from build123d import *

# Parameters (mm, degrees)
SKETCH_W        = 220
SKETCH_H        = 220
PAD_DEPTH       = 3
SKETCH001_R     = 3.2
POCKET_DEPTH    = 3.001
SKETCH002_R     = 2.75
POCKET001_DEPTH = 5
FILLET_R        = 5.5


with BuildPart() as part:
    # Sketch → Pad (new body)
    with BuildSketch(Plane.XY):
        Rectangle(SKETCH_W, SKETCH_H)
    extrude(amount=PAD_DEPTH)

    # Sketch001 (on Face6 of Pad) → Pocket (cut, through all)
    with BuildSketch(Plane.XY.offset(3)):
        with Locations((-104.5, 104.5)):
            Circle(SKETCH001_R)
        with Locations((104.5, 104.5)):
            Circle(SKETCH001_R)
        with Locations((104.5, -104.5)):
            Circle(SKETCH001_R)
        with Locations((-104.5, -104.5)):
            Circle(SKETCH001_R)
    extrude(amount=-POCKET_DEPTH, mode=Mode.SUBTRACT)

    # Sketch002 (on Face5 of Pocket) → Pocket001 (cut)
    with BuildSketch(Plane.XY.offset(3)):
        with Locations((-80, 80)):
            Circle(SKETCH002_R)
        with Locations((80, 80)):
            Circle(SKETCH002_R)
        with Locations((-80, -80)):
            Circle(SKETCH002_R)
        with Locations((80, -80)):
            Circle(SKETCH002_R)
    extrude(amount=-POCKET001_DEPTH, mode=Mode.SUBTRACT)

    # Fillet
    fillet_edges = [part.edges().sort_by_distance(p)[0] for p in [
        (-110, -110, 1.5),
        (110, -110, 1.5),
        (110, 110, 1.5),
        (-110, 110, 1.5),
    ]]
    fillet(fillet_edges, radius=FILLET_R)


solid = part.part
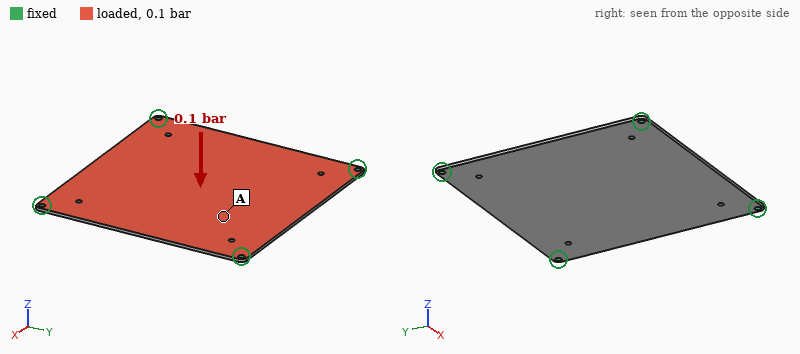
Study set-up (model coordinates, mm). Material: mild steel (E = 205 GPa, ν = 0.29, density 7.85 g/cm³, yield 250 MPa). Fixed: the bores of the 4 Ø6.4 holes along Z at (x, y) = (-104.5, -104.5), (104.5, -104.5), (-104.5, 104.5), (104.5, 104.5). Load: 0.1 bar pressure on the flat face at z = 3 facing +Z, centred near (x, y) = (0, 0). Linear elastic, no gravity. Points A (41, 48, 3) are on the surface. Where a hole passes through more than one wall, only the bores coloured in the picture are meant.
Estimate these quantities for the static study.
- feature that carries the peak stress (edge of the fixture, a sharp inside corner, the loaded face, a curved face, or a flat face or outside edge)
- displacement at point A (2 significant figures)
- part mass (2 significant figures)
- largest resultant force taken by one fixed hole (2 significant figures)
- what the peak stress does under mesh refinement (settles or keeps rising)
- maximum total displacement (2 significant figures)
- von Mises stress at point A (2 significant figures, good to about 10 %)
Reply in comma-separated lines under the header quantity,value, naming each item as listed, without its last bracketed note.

quantity,value
feature that carries the peak stress,edge of the fixture
displacement at point A,0.28 mm
part mass,1.1 kg
largest resultant force taken by one fixed hole,120 N
what the peak stress does under mesh refinement,keeps rising
maximum total displacement,0.37 mm
von Mises stress at point A,14 MPa
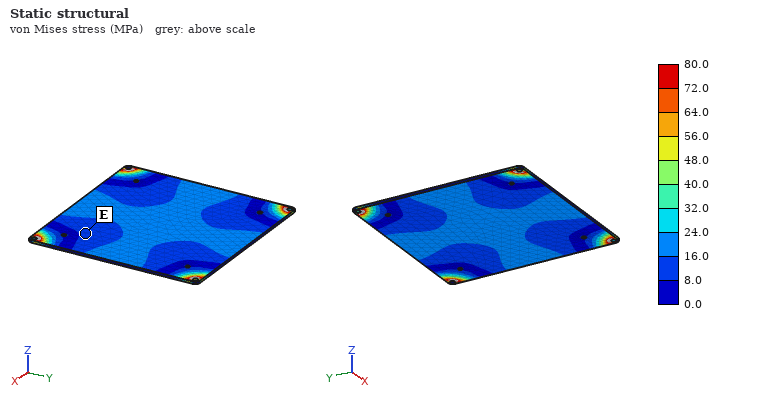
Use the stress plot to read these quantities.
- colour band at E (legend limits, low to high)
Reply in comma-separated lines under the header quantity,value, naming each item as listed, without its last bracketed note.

quantity,value
colour band at E,8.0 to 16.0 MPa
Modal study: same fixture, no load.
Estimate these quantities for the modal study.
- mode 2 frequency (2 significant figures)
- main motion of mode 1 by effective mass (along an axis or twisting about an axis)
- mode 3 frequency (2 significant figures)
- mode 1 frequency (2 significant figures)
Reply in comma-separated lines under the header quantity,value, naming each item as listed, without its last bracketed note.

quantity,value
mode 2 frequency,380 Hz
main motion of mode 1 by effective mass,along Z
mode 3 frequency,380 Hz
mode 1 frequency,200 Hz
